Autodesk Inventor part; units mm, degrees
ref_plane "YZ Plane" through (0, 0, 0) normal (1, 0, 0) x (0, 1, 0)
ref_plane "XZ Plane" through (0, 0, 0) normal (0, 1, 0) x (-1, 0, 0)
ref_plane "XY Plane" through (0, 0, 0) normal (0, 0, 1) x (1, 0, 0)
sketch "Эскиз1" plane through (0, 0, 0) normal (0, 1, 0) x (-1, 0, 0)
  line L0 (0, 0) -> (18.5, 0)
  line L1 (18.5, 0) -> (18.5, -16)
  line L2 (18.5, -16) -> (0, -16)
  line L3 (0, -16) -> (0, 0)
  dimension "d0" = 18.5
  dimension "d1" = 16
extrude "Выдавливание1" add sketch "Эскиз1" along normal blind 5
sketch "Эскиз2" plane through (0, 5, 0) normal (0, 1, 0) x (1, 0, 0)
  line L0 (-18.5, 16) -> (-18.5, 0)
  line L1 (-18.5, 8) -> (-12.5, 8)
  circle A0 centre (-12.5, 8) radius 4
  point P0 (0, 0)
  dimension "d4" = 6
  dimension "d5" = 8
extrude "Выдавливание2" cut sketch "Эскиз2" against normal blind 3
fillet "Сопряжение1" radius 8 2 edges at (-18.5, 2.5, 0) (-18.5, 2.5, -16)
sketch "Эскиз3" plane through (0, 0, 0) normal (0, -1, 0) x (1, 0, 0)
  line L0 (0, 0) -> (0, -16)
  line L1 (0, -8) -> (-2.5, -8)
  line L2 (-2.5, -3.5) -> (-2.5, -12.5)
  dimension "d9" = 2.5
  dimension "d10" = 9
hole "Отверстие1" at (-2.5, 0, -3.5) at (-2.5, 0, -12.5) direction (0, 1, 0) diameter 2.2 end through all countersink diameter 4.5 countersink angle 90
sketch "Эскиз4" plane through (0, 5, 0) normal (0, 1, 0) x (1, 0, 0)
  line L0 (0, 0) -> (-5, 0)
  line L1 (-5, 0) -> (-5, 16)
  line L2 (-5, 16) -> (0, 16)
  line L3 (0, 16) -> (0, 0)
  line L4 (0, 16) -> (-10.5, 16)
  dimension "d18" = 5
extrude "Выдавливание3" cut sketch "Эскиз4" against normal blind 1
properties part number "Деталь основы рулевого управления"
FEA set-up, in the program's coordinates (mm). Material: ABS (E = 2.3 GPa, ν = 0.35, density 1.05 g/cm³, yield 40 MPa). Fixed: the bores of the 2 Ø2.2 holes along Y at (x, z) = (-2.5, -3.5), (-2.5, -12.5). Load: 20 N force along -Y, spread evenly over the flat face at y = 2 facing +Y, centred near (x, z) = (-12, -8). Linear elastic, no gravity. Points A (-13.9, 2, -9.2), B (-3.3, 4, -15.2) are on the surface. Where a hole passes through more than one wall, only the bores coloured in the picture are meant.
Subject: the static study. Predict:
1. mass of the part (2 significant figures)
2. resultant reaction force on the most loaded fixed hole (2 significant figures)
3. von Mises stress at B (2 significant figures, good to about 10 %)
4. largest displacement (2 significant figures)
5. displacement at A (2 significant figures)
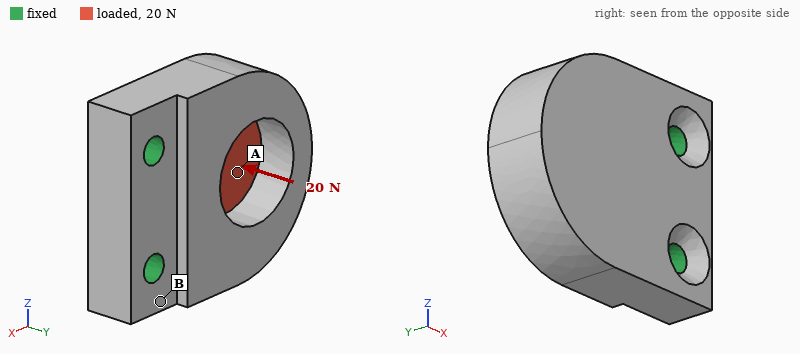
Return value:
1.1 g
10 N
3.1 MPa
93 µm
63 µm
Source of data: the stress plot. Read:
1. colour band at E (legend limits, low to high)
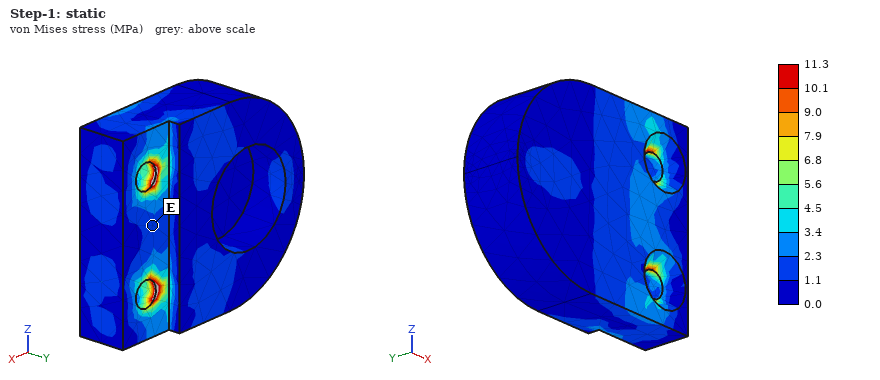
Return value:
1.1 to 2.3 MPa
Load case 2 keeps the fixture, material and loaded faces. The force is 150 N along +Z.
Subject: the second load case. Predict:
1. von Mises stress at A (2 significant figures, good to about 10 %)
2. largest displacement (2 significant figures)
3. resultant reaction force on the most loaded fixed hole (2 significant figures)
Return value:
6.2 MPa
92 µm
160 N
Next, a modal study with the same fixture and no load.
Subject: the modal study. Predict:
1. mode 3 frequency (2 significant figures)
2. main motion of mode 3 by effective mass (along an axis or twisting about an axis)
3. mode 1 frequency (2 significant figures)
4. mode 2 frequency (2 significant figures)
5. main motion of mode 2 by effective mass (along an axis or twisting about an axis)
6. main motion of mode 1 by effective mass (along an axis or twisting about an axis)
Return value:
9800 Hz
along Z
3700 Hz
8500 Hz
along Z
along Y
